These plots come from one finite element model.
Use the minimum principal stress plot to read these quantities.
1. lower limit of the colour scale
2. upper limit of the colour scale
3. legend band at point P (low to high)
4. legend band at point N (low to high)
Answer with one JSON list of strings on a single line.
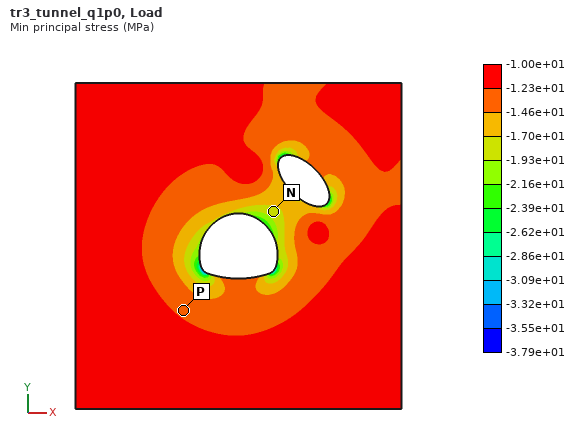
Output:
["-3.79e+01 MPa", "-1.00e+01 MPa", "-1.46e+01 to -1.23e+01 MPa", "-1.93e+01 to -1.70e+01 MPa"]
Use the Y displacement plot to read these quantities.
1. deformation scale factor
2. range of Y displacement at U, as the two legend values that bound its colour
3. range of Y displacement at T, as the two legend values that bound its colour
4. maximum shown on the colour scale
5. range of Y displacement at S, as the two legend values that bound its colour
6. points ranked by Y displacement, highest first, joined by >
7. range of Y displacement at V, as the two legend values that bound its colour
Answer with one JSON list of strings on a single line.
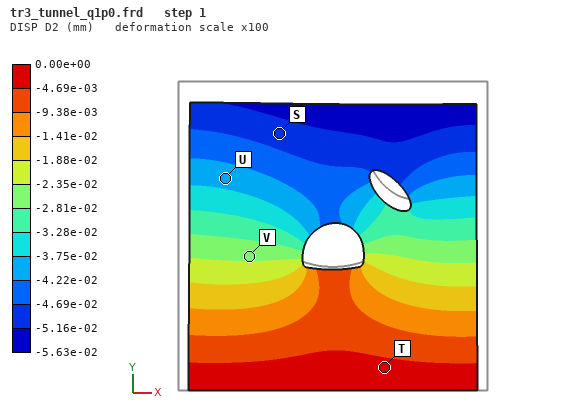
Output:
["100", "-4.22e-02 to -3.75e-02 mm", "-4.69e-03 to 0.00e+00 mm", "0.00e+00 mm", "-5.16e-02 to -4.69e-02 mm", "T > V > U > S", "-2.81e-02 to -2.35e-02 mm"]
